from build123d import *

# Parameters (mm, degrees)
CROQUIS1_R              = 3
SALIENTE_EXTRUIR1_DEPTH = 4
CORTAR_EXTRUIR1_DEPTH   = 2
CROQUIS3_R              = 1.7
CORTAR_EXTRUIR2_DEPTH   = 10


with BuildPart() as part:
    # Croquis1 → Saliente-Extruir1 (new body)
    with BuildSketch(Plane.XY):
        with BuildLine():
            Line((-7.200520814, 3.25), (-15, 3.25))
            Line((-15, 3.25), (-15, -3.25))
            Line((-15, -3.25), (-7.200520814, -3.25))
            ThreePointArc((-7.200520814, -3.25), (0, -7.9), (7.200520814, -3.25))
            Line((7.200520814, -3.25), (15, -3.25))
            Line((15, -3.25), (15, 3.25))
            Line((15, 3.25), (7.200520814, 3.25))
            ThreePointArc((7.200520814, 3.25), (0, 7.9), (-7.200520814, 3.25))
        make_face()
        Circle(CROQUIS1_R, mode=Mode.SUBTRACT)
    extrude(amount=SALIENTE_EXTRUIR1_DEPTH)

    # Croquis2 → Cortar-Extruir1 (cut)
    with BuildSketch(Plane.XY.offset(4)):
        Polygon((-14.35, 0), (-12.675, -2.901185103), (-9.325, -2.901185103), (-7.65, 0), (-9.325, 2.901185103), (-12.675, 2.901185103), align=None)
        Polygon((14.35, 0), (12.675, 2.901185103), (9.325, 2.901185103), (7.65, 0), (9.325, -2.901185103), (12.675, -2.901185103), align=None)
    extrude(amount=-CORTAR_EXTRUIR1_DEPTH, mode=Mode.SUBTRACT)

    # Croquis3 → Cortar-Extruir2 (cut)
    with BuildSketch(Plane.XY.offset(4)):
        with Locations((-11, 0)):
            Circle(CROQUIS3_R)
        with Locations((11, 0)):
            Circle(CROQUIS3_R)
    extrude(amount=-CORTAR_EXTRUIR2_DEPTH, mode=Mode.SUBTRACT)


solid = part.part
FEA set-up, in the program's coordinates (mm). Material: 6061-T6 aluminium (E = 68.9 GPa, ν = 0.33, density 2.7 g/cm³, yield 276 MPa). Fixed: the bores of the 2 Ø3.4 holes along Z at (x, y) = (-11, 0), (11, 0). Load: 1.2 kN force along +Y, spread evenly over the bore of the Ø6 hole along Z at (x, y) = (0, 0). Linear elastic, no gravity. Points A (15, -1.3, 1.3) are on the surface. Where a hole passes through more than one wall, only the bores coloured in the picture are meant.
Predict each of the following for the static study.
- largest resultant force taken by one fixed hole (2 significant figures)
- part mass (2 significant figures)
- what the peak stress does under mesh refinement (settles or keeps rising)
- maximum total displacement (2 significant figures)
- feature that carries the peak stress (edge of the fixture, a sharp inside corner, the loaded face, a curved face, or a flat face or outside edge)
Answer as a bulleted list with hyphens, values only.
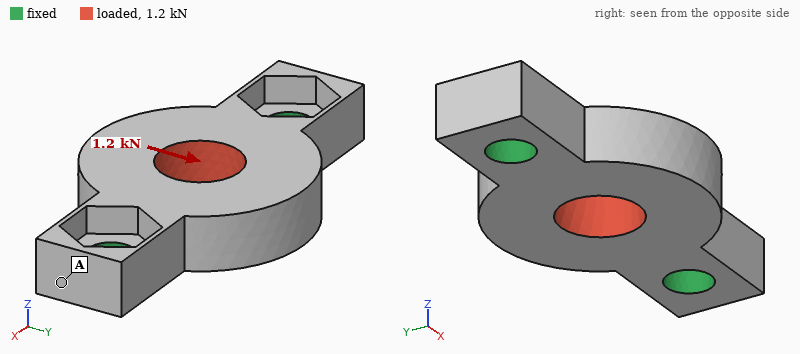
- 600 N
- 2.4 g
- keeps rising
- 22 µm
- edge of the fixture
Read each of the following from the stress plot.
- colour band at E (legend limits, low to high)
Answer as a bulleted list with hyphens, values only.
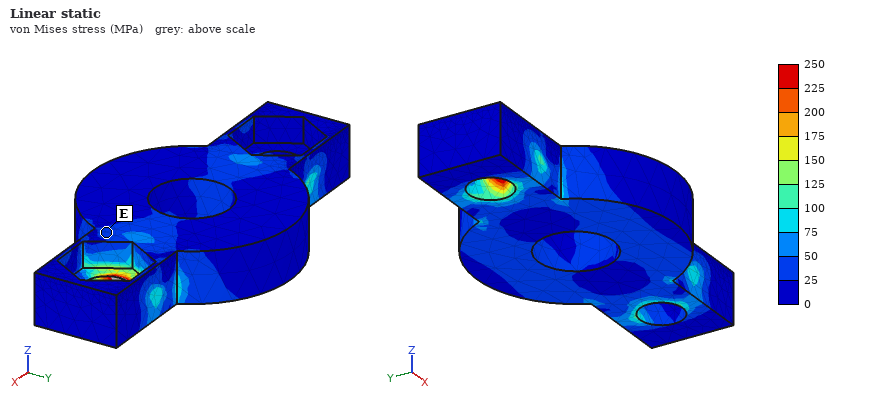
- 25 to 50 MPa
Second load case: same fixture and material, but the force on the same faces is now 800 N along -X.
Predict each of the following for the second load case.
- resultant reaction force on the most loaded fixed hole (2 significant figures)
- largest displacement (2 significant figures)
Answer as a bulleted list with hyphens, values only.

- 400 N
- 2.9 µm
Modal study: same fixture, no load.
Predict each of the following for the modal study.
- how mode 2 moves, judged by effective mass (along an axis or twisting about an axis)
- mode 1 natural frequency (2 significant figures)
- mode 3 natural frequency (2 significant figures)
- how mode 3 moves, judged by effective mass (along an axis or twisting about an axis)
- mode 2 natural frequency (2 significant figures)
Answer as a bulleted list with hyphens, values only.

- along Z
- 18 kHz
- 45 kHz
- along Y
- 24 kHz
